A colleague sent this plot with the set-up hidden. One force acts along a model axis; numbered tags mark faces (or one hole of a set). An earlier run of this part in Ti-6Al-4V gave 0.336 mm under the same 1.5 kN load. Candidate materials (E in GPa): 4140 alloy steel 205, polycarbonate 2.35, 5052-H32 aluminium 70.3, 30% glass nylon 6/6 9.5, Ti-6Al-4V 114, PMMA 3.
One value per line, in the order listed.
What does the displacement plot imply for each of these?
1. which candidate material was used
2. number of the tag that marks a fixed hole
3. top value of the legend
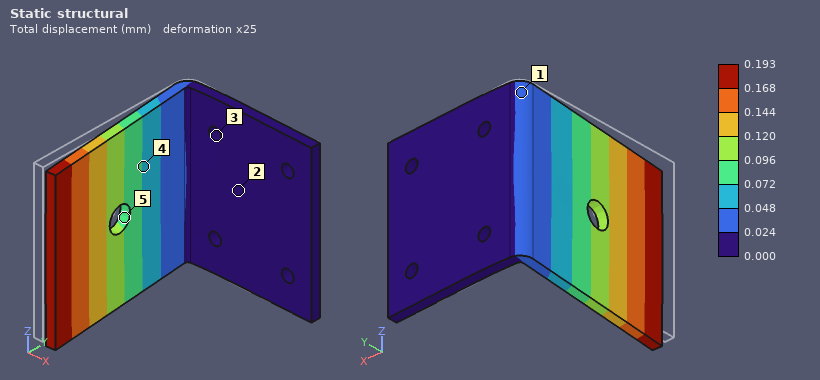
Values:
4140 alloy steel
3
0.193 mm
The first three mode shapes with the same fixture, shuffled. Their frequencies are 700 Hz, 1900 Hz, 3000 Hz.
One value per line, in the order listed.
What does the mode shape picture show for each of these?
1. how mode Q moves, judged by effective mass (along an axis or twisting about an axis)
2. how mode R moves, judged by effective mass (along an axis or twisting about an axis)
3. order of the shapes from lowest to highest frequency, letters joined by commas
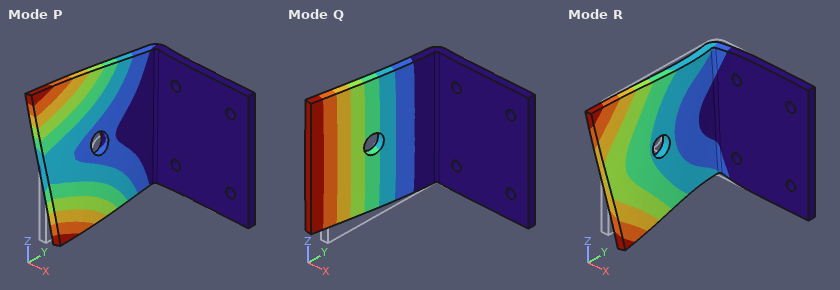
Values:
along X
along Z
Q, P, R
